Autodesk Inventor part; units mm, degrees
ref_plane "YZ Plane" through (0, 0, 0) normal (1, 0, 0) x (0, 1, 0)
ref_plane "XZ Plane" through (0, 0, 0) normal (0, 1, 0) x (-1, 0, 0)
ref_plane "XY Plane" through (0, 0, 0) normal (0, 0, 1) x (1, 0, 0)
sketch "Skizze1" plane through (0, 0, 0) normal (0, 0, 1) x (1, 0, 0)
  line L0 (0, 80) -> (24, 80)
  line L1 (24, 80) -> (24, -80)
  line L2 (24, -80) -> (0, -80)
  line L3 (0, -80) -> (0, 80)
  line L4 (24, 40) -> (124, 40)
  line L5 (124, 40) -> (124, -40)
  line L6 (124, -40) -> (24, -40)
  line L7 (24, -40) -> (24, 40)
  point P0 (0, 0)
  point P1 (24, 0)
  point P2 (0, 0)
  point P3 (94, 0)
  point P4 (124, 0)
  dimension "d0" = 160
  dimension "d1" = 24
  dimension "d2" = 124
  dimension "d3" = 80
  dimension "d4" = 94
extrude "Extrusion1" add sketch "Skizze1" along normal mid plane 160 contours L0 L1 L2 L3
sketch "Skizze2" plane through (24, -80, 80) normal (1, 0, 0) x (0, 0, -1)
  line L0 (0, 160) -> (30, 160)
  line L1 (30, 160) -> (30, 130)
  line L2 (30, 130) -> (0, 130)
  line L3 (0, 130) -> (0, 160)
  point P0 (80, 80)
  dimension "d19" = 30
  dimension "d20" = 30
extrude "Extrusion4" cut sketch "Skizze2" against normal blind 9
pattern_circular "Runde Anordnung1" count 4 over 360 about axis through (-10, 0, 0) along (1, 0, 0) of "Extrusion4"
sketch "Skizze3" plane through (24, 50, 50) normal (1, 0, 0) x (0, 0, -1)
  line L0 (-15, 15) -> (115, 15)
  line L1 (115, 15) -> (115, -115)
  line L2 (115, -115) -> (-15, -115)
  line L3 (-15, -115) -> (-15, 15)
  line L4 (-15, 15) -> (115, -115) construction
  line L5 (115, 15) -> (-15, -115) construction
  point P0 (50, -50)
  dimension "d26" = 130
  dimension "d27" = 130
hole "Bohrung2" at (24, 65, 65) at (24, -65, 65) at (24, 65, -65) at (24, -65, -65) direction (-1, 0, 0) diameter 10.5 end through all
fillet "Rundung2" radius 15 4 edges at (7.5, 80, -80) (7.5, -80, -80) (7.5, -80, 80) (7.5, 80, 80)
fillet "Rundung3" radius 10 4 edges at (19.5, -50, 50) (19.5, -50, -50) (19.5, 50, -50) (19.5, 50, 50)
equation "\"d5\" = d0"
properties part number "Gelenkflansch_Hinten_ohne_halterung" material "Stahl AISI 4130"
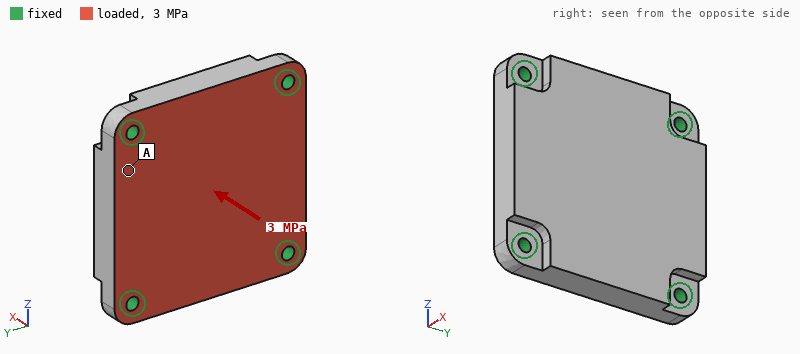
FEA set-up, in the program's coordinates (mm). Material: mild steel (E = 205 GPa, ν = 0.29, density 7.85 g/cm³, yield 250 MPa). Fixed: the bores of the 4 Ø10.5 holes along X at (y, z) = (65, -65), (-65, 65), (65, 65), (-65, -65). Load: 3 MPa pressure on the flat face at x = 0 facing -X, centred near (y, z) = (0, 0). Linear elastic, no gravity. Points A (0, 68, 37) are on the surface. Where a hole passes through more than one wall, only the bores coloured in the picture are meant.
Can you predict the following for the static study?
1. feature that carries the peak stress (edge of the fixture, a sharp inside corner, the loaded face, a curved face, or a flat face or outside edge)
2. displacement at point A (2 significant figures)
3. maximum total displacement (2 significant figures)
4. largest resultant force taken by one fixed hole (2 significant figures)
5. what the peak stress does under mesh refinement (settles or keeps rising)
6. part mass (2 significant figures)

edge of the fixture
18 µm
46 µm
21 kN
keeps rising
4.5 kg
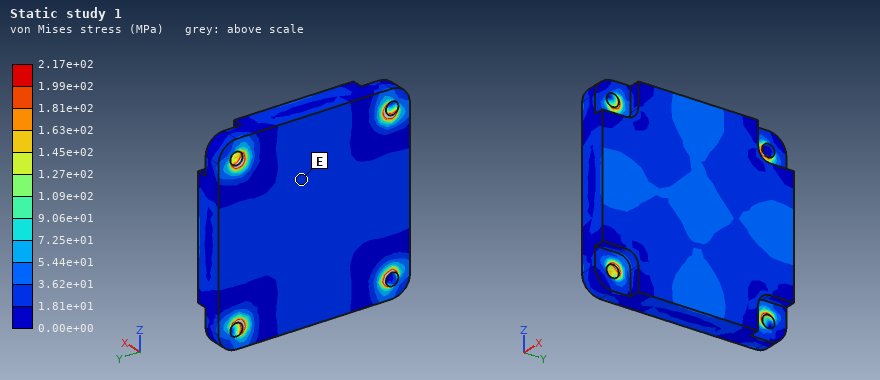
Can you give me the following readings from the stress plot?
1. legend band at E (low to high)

1.81e+01 to 3.62e+01 MPa
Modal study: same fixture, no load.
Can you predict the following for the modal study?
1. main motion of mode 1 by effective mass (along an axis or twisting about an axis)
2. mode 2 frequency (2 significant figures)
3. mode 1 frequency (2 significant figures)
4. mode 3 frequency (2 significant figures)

along X
5600 Hz
3500 Hz
5600 Hz
